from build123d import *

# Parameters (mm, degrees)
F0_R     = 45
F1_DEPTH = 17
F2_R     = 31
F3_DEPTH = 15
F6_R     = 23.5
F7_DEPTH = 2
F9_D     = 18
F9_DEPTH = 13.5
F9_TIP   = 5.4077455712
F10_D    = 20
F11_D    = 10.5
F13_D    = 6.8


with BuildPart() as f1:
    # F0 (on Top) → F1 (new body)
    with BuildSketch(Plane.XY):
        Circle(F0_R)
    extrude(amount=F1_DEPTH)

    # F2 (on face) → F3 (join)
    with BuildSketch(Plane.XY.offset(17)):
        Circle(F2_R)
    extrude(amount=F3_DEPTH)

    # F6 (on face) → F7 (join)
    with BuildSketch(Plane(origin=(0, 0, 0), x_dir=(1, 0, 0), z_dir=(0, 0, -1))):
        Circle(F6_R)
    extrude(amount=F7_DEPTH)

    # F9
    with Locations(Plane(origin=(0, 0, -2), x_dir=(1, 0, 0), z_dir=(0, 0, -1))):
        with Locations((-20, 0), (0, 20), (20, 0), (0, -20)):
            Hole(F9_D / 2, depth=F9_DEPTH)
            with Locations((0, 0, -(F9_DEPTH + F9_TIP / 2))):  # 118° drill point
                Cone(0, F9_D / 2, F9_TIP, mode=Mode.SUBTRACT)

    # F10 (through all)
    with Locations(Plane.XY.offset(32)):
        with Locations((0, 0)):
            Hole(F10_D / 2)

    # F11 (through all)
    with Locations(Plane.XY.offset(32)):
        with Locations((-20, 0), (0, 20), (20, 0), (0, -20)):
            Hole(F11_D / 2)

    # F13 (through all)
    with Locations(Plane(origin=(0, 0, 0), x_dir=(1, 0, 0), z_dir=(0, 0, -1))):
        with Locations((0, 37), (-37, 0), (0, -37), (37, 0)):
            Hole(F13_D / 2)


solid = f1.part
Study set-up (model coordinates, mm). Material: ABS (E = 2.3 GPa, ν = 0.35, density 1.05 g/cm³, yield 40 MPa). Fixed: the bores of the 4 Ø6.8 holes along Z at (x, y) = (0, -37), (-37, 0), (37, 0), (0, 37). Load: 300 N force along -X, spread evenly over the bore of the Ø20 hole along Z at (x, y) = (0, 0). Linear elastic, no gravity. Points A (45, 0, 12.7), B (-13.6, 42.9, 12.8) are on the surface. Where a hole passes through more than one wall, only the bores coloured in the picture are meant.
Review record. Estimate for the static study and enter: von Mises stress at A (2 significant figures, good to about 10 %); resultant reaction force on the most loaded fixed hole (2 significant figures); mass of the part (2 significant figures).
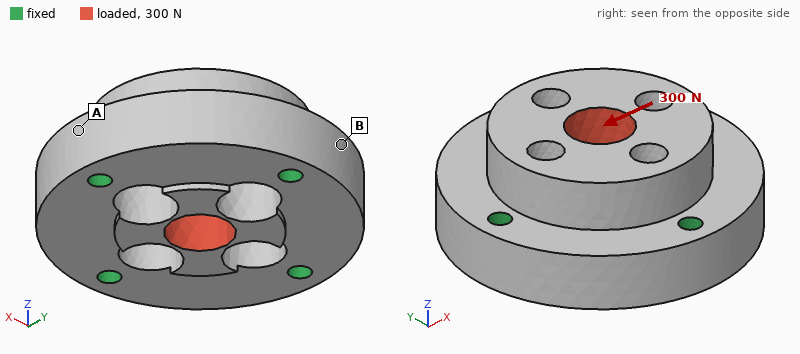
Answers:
0.20 MPa
87 N
130 g
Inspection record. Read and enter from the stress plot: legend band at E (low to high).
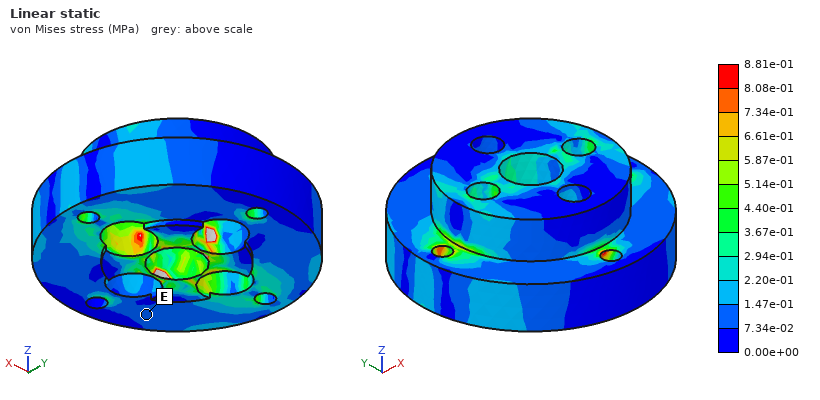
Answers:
7.34e-02 to 1.47e-01 MPa
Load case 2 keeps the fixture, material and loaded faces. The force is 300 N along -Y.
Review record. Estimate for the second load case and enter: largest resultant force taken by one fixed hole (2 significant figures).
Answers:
87 N
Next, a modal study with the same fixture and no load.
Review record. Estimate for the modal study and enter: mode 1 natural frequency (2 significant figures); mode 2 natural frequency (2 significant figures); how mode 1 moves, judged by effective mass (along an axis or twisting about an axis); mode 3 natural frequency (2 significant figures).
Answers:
4500 Hz
4900 Hz
along Z
4900 Hz
